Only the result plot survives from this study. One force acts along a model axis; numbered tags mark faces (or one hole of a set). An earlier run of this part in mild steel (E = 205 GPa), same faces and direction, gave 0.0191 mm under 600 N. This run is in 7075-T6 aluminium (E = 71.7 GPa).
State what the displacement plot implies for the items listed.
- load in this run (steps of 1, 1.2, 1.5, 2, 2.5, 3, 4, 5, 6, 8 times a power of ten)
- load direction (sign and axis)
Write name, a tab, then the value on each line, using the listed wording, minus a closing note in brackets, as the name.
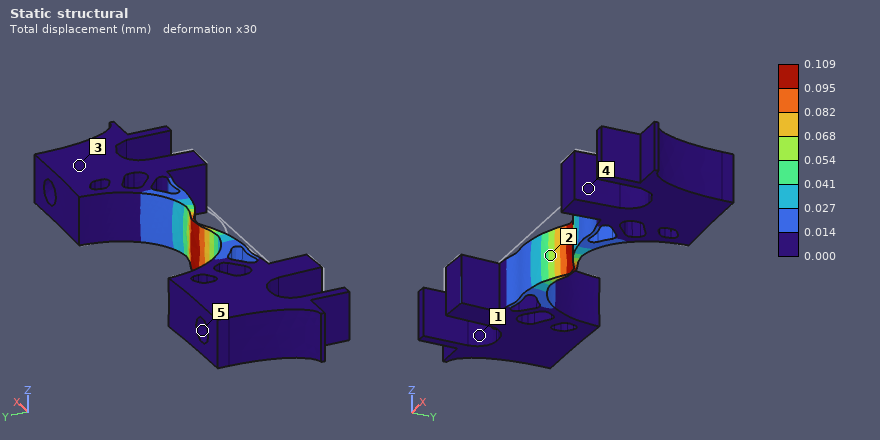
load in this run	1.2 kN
load direction	+Y
